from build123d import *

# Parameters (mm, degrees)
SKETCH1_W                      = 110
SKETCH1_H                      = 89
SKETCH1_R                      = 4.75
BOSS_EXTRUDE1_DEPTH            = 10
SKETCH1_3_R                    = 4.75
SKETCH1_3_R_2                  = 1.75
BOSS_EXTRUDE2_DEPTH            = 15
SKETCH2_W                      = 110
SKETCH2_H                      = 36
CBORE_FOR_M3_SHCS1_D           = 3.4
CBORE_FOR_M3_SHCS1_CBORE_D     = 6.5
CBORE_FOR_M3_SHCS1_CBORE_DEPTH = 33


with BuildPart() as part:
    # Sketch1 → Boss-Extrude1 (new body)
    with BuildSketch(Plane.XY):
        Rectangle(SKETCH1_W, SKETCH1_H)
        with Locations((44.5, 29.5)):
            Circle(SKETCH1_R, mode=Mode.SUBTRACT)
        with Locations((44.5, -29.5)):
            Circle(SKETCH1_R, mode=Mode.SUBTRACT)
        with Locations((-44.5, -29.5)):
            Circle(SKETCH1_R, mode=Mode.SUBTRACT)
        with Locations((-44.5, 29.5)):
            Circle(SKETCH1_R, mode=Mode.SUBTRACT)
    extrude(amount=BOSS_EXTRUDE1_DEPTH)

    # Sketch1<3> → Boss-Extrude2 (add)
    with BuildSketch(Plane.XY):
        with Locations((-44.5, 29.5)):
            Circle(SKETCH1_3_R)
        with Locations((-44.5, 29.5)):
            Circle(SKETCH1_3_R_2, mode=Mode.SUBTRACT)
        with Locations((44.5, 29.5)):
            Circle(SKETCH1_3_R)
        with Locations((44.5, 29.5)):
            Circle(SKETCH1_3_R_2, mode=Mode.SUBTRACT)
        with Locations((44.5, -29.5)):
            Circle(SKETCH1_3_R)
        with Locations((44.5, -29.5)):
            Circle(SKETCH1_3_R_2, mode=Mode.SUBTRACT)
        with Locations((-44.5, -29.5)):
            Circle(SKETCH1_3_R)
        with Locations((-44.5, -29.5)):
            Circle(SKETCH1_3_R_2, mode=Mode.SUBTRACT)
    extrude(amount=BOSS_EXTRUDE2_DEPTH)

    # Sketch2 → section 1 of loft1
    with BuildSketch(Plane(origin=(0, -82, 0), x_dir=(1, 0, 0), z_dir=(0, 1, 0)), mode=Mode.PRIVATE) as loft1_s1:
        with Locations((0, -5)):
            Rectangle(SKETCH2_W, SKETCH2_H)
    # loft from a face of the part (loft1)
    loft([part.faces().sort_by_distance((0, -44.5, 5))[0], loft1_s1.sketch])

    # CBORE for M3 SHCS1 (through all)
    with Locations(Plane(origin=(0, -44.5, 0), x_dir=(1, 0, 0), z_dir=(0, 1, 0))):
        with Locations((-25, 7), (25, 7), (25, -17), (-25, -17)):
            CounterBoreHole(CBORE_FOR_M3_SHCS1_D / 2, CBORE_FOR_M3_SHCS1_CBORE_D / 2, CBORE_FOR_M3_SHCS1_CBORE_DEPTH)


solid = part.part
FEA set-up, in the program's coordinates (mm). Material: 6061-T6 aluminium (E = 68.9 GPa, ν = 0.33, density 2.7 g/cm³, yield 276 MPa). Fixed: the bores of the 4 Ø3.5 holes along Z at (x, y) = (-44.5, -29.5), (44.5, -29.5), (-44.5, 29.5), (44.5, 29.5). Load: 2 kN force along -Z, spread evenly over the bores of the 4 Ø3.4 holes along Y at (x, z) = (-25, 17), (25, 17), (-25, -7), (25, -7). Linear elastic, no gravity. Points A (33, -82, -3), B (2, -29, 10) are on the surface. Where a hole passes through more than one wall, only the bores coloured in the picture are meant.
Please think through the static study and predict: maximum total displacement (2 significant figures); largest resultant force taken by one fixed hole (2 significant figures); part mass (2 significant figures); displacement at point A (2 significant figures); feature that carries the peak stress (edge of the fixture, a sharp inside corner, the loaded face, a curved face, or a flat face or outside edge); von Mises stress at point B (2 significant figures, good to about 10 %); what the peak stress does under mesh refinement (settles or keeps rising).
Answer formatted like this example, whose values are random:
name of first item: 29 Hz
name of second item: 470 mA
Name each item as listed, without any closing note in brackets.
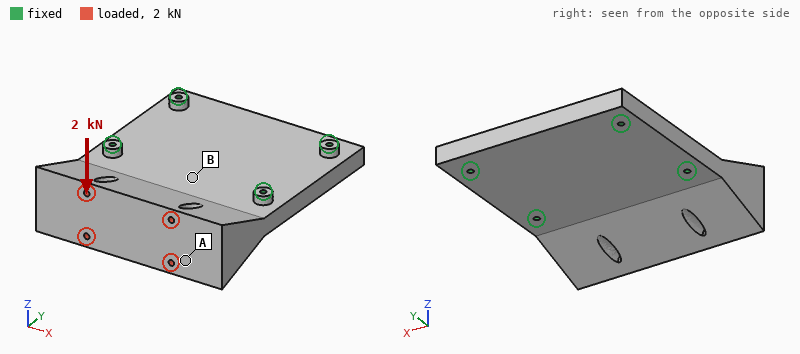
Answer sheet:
maximum total displacement: 0.18 mm
largest resultant force taken by one fixed hole: 1.4 kN
part mass: 520 g
displacement at point A: 0.17 mm
feature that carries the peak stress: edge of the fixture
von Mises stress at point B: 25 MPa
what the peak stress does under mesh refinement: keeps rising
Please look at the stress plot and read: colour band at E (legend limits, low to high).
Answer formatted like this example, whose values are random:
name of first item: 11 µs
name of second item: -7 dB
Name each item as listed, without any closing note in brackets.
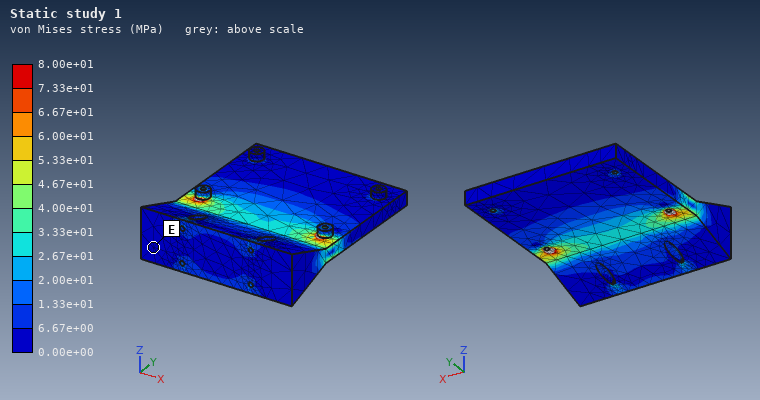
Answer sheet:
colour band at E: 0.00e+00 to 6.67e+00 MPa
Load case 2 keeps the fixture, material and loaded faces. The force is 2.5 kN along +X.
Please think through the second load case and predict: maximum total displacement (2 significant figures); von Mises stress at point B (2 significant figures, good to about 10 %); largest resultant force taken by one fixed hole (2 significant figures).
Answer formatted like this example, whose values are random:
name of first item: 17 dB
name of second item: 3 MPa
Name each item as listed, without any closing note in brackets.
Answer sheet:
maximum total displacement: 7.5 µm
von Mises stress at point B: 2.1 MPa
largest resultant force taken by one fixed hole: 1.7 kN
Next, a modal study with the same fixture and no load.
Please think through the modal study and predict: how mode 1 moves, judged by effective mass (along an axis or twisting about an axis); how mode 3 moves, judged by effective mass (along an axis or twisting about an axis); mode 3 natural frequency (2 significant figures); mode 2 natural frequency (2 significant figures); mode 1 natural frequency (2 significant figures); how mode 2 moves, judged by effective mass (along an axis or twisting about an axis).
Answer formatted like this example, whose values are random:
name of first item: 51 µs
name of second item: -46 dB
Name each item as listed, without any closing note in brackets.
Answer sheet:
how mode 1 moves, judged by effective mass: along Z
how mode 3 moves, judged by effective mass: along Z
mode 3 natural frequency: 5200 Hz
mode 2 natural frequency: 4000 Hz
mode 1 natural frequency: 1500 Hz
how mode 2 moves, judged by effective mass: twisting about Y
